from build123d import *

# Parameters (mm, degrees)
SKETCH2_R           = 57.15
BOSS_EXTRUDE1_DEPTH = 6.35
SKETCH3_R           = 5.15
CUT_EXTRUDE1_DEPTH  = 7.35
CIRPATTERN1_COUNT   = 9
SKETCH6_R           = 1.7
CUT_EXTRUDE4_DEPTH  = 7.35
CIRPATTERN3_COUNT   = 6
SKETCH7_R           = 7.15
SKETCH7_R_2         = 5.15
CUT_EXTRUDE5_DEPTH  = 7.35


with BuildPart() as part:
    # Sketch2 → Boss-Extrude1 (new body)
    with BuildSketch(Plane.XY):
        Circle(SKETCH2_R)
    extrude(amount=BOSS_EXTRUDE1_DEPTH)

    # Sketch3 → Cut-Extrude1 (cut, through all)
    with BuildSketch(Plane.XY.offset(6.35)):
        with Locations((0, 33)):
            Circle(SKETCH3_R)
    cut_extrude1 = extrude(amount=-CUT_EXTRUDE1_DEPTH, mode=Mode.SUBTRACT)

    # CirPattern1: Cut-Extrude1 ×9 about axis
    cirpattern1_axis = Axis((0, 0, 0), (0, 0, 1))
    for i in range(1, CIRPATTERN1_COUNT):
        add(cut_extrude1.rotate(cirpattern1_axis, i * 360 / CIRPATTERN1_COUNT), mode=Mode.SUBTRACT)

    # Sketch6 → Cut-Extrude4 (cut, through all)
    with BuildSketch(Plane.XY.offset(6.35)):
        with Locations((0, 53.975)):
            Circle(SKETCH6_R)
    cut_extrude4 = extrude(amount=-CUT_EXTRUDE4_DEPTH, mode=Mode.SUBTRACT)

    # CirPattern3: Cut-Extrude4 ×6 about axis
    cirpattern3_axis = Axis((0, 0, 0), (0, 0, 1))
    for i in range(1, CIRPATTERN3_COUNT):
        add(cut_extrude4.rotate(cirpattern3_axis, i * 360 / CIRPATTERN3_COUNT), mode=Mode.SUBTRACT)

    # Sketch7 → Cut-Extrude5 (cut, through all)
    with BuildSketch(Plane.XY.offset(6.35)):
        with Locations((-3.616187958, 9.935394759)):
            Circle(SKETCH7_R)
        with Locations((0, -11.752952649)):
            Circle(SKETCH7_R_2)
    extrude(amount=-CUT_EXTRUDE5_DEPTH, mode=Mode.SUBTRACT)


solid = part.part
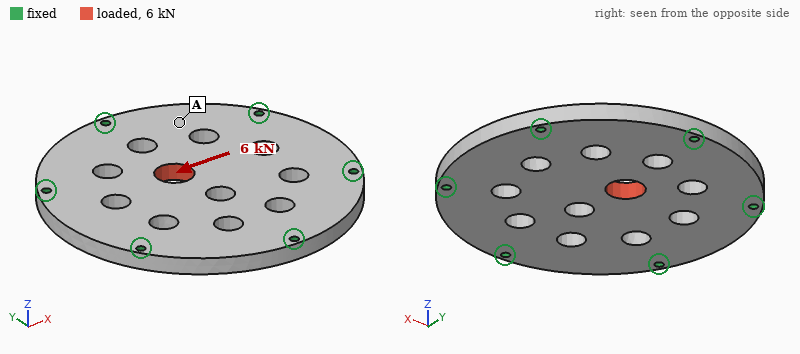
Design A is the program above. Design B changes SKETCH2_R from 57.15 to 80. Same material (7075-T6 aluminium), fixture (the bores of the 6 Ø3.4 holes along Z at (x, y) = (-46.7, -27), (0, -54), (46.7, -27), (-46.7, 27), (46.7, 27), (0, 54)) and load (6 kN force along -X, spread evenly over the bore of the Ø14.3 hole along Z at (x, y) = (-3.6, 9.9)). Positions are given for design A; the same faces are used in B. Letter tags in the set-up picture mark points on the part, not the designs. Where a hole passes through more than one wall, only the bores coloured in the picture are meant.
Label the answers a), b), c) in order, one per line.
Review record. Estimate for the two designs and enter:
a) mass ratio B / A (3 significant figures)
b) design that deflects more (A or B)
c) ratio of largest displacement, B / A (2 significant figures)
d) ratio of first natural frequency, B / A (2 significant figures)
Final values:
a) 2.07
b) A
c) 0.87
d) 0.94
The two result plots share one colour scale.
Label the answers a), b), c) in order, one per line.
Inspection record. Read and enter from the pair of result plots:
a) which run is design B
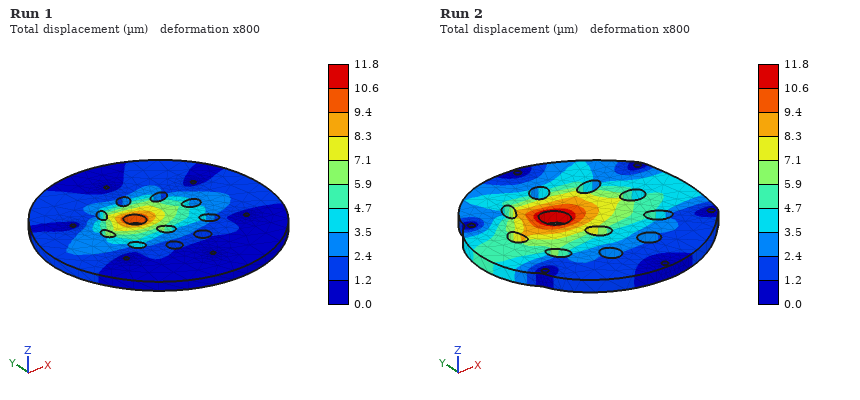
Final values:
a) Run 1
